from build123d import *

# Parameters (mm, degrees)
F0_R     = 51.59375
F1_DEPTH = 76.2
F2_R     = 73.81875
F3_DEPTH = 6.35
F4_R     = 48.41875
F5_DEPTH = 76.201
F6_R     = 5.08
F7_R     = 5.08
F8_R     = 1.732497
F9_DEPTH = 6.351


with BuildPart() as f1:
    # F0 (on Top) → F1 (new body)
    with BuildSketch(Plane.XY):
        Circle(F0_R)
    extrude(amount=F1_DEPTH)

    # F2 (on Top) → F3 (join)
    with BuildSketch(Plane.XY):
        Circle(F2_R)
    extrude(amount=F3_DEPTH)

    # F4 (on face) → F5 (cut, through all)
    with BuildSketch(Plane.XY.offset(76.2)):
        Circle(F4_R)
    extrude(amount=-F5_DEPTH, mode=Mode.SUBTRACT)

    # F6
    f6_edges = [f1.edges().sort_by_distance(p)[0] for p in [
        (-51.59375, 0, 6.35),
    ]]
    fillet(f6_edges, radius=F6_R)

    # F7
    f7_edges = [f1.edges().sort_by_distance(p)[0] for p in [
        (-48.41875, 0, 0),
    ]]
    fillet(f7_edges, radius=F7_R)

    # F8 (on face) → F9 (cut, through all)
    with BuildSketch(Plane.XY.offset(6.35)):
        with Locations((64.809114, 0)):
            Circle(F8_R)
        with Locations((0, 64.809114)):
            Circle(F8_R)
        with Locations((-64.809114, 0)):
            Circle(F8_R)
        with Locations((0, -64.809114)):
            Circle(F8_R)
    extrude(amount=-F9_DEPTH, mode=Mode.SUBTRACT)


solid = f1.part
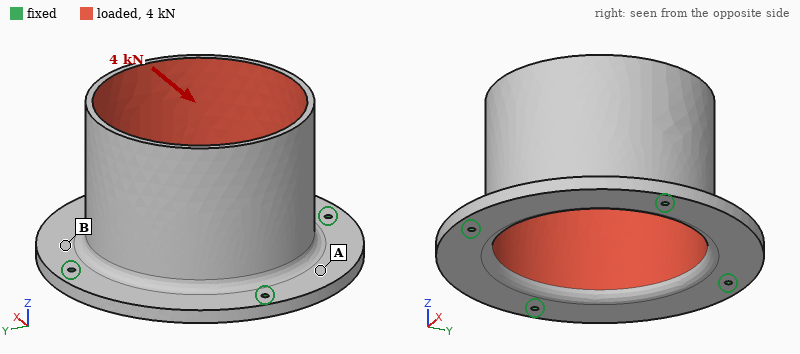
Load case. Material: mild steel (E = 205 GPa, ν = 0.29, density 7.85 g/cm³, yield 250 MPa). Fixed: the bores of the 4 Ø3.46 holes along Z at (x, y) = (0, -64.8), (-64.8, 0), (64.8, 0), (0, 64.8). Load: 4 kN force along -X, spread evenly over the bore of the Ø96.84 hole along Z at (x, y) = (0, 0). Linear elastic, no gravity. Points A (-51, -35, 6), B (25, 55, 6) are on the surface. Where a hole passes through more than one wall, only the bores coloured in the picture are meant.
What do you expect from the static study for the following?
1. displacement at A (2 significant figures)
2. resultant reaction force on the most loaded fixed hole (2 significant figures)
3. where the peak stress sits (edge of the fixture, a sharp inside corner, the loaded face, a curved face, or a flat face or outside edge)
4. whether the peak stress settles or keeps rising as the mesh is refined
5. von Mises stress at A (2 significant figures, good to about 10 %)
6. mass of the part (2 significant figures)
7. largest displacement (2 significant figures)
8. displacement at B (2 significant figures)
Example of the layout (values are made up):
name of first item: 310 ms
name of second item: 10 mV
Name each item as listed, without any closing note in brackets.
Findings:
displacement at A: 8.3 µm
resultant reaction force on the most loaded fixed hole: 1.5 kN
where the peak stress sits: edge of the fixture
whether the peak stress settles or keeps rising as the mesh is refined: keeps rising
von Mises stress at A: 11 MPa
mass of the part: 1.0 kg
largest displacement: 22 µm
displacement at B: 5.7 µm
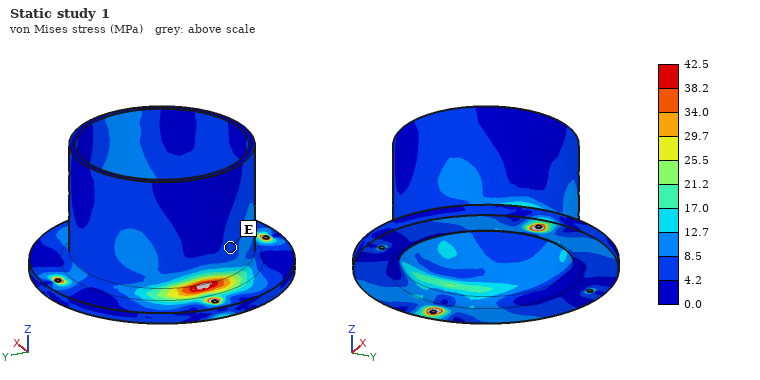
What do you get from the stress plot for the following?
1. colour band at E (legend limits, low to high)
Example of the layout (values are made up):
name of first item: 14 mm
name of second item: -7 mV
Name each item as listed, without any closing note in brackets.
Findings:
colour band at E: 4.2 to 8.5 MPa
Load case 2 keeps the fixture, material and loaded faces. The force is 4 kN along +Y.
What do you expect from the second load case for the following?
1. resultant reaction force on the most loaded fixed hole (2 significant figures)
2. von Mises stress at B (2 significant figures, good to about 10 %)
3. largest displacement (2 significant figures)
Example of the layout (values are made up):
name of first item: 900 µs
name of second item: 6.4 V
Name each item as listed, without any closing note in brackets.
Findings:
resultant reaction force on the most loaded fixed hole: 1.5 kN
von Mises stress at B: 14 MPa
largest displacement: 22 µm
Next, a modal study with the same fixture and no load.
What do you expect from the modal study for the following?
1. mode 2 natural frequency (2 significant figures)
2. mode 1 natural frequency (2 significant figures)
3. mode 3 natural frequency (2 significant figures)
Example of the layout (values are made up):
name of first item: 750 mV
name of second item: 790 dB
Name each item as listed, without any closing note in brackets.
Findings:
mode 2 natural frequency: 2500 Hz
mode 1 natural frequency: 1400 Hz
mode 3 natural frequency: 2500 Hz
